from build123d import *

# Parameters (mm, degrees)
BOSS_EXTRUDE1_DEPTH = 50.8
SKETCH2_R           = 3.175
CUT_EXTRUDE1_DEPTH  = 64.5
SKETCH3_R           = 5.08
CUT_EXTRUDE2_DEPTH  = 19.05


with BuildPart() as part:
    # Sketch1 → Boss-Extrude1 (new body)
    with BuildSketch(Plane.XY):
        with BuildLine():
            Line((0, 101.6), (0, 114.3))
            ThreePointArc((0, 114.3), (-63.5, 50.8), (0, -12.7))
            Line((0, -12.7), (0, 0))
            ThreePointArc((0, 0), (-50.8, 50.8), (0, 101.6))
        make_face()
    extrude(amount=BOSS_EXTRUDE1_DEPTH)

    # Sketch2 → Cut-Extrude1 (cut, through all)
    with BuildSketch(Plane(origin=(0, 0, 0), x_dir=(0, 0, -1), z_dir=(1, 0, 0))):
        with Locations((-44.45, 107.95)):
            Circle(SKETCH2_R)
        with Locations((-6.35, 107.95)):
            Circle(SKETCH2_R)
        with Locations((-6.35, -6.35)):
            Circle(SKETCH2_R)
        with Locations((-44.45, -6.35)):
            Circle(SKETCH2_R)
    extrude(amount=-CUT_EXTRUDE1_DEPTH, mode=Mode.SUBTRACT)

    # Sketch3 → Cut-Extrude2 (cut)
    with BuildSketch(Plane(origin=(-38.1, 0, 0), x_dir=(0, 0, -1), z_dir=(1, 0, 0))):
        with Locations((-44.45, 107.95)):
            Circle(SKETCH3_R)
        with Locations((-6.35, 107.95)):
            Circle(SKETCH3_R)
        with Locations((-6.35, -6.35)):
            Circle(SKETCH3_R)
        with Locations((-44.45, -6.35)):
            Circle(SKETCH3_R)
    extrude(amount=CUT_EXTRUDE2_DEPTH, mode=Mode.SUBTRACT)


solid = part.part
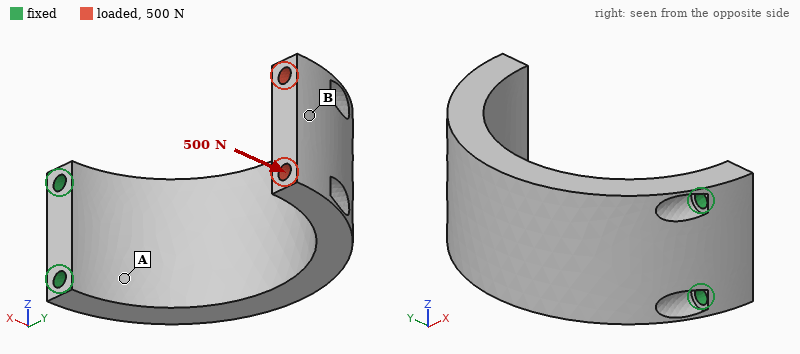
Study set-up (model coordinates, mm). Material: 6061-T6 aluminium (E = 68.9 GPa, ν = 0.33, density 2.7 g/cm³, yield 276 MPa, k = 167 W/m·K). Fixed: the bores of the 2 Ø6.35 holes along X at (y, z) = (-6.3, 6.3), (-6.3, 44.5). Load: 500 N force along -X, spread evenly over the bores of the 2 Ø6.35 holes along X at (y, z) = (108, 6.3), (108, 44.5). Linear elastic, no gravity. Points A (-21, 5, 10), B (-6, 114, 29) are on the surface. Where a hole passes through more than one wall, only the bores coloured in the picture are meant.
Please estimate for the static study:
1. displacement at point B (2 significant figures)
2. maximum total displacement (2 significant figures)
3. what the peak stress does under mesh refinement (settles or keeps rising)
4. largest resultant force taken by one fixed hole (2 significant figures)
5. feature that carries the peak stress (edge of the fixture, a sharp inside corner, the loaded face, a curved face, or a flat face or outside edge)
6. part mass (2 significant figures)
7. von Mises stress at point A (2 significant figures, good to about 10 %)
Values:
0.80 mm
0.83 mm
keeps rising
250 N
edge of the fixture
300 g
50 MPa
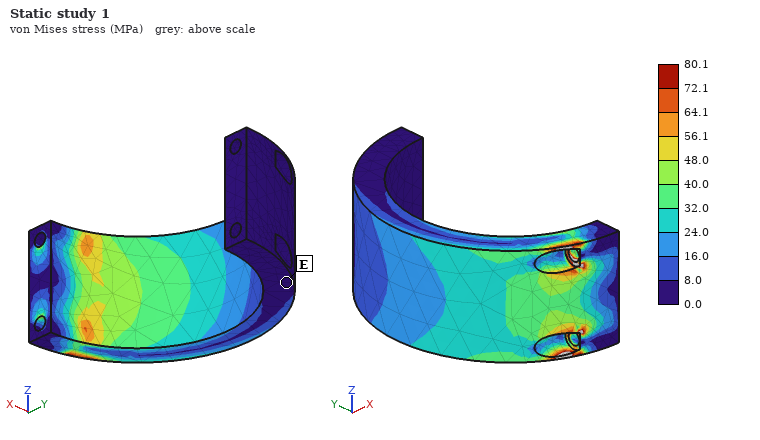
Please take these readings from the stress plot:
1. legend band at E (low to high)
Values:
0.0 to 8.0 MPa
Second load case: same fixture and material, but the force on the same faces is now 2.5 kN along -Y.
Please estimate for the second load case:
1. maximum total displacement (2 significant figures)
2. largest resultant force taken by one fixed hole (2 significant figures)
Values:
1.6 mm
1.3 kN
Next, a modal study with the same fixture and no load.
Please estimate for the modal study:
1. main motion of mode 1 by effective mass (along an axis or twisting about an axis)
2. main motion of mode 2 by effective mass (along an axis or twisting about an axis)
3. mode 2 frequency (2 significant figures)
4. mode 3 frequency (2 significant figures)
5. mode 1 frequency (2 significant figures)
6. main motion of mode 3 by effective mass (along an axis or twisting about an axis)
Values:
along X
along Z
690 Hz
1400 Hz
410 Hz
along Y
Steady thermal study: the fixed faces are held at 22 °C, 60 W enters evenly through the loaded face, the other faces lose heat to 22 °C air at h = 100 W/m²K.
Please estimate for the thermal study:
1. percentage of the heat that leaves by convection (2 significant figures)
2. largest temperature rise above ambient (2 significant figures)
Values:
72 %
47 K
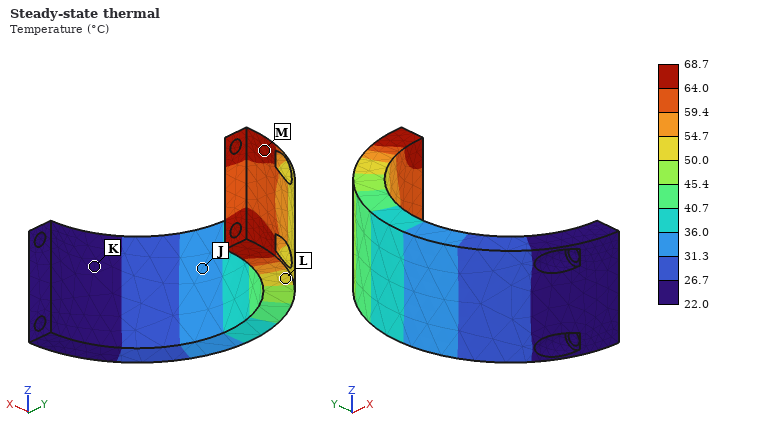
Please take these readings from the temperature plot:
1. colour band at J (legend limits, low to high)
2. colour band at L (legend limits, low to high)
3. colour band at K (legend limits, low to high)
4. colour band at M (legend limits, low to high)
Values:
31.3 to 36.0 °C
50.0 to 54.7 °C
22.0 to 26.7 °C
64.0 to 68.7 °C
